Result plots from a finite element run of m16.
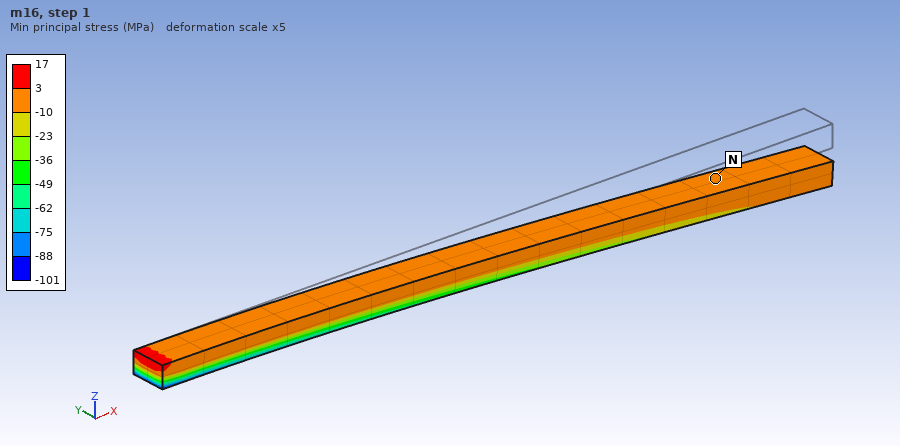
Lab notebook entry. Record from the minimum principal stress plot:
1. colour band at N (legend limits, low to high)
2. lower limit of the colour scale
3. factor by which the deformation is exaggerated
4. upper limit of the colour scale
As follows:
-10 to 3 MPa
-101 MPa
5
17 MPa
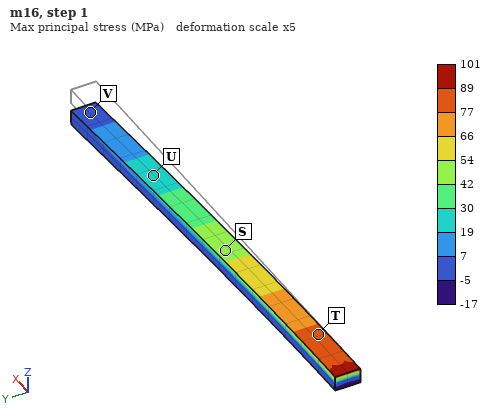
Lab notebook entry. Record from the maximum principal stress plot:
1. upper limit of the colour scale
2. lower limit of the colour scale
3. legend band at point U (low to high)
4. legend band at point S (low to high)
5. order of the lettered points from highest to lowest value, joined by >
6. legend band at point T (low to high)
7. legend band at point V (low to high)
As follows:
101 MPa
-17 MPa
19 to 30 MPa
42 to 54 MPa
T > S > U > V
77 to 89 MPa
-5 to 7 MPa
